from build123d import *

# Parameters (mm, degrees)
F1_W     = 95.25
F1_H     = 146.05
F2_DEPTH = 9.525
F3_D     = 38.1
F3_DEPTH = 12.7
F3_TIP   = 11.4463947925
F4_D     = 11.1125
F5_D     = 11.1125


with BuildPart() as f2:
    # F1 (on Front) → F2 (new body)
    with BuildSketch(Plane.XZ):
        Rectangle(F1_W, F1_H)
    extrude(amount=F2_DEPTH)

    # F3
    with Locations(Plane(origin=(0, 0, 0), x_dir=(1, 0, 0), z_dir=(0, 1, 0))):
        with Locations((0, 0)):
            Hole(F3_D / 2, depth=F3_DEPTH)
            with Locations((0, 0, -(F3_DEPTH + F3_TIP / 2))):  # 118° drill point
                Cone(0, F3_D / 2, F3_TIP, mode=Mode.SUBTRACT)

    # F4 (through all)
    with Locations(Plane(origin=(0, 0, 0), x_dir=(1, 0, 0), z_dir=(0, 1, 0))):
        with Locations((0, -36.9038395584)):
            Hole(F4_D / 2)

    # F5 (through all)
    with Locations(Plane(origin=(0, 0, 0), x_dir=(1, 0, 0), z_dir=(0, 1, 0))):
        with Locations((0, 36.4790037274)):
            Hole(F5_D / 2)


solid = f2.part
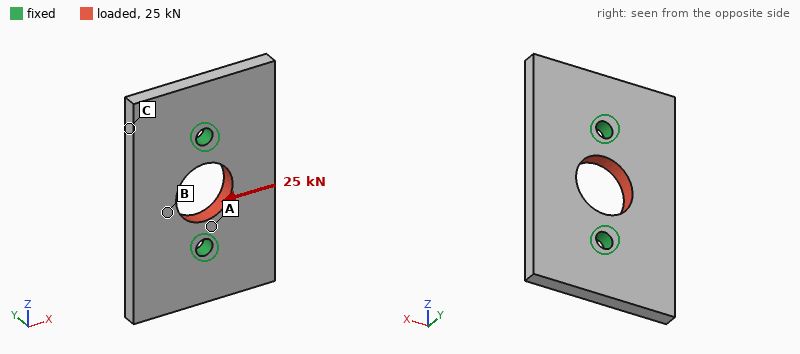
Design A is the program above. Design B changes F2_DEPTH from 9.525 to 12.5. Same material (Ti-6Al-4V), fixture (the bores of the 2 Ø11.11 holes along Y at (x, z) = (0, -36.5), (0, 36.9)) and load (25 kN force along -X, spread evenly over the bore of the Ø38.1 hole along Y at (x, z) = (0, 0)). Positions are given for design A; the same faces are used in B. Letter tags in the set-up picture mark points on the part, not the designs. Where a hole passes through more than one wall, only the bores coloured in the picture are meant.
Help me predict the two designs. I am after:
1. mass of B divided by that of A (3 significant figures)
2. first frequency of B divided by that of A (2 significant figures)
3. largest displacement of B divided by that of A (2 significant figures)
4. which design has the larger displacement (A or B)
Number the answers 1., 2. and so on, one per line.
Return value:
1. 1.31
2. 1.2
3. 0.76
4. A
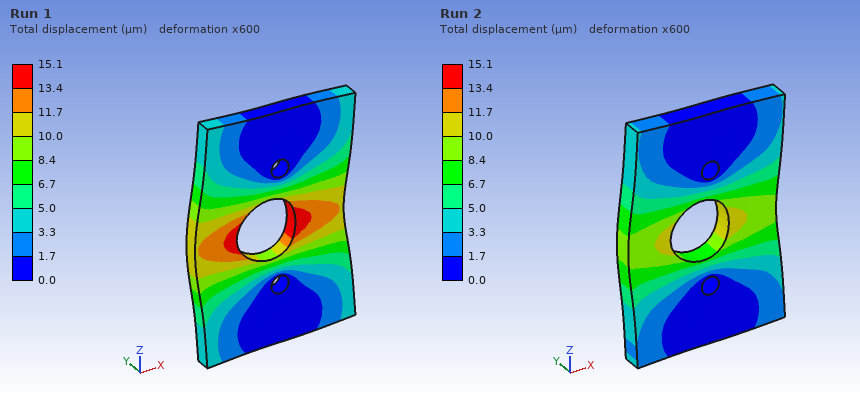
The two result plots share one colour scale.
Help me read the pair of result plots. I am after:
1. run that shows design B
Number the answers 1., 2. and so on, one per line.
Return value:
1. Run 2
